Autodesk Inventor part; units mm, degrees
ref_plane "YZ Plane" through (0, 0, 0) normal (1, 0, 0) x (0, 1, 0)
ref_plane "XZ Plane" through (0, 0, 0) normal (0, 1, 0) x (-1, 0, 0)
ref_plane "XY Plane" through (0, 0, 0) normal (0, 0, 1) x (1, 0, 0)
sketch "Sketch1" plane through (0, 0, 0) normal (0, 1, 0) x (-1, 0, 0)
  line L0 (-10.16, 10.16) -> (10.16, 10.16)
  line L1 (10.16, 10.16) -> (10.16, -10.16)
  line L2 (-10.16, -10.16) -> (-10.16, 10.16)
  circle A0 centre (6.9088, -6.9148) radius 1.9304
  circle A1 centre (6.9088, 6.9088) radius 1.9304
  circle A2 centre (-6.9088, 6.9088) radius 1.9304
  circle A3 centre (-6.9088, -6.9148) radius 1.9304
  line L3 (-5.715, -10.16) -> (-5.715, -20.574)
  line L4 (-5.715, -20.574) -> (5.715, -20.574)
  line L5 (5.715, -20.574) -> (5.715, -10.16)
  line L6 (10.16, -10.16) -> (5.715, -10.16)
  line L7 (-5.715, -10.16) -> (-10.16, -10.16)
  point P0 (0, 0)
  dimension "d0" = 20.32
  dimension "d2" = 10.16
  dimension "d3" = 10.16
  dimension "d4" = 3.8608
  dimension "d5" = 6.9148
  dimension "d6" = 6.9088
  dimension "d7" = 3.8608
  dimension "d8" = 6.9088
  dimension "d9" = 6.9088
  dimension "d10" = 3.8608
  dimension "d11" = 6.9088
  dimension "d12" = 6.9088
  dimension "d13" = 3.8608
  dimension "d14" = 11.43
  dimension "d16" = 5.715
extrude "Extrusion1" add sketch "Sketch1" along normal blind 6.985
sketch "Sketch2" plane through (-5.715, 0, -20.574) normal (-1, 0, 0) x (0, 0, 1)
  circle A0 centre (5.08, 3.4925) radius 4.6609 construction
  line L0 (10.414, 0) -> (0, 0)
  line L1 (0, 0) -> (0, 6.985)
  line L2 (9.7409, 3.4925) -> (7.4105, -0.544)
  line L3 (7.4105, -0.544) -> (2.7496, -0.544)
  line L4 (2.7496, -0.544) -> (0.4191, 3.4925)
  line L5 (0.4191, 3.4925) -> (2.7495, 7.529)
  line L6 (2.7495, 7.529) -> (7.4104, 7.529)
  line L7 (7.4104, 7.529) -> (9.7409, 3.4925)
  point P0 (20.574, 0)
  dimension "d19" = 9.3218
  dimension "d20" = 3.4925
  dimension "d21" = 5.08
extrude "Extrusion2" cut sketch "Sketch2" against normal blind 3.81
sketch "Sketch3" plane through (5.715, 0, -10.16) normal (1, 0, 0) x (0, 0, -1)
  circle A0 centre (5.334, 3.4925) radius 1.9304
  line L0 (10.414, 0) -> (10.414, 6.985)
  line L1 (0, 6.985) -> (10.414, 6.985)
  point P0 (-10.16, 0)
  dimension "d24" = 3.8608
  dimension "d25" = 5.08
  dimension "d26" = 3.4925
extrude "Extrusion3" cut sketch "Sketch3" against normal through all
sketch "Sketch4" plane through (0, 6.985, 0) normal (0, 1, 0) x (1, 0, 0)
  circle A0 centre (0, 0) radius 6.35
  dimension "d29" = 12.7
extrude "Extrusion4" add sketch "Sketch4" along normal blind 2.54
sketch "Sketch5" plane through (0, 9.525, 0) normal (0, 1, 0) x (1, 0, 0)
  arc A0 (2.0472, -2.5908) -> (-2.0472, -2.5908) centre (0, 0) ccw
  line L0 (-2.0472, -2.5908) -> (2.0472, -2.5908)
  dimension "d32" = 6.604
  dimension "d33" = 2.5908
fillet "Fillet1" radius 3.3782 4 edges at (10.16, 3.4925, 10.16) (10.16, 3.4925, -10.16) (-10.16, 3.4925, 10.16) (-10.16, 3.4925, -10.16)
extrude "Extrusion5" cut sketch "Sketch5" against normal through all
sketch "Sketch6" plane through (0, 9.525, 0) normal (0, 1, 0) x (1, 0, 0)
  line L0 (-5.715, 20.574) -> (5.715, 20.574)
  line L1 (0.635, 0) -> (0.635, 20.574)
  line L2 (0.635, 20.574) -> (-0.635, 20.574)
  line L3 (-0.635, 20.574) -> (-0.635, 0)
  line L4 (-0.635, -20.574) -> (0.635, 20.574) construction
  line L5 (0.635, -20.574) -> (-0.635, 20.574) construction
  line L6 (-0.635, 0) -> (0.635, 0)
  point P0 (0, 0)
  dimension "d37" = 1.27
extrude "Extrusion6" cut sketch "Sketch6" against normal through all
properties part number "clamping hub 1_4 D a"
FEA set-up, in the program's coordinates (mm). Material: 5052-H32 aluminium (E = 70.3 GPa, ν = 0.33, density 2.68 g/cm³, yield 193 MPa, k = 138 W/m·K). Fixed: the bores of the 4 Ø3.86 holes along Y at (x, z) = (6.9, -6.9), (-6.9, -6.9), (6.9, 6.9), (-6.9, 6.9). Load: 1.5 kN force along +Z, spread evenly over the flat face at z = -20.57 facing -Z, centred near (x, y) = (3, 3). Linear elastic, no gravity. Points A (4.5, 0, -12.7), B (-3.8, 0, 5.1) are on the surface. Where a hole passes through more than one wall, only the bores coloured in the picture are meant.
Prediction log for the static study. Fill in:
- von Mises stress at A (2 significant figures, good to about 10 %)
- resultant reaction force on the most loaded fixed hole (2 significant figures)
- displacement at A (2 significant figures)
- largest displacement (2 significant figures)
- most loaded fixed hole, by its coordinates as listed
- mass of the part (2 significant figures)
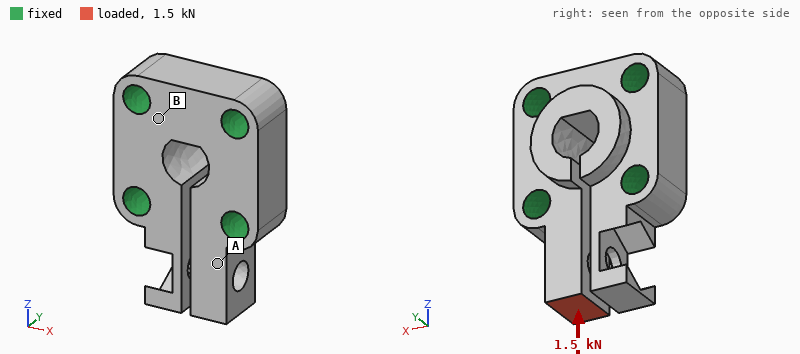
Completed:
81 MPa
1.3 kN
7.2 µm
23 µm
(6.9, -6.9)
7.8 g
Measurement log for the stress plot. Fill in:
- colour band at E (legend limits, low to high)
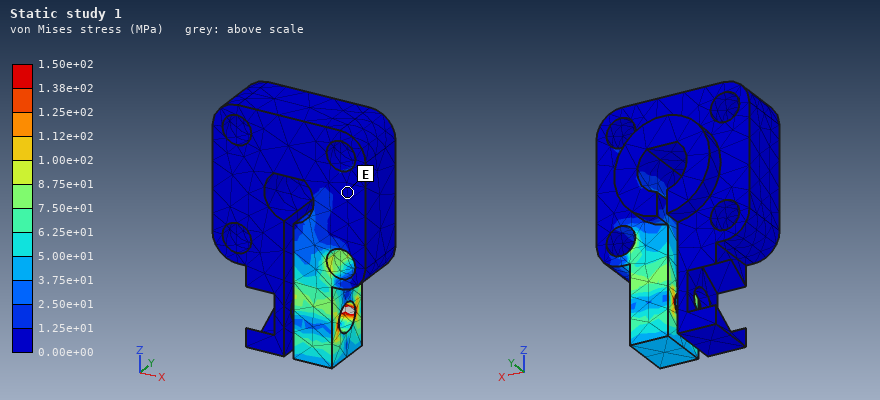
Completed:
0.00e+00 to 1.25e+01 MPa
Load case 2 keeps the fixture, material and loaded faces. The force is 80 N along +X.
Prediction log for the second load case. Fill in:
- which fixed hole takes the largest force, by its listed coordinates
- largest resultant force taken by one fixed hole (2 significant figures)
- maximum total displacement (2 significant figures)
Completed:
(6.9, -6.9)
130 N
16 µm
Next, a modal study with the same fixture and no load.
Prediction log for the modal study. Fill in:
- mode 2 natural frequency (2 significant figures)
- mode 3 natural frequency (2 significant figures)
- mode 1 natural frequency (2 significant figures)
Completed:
14 kHz
22 kHz
6300 Hz
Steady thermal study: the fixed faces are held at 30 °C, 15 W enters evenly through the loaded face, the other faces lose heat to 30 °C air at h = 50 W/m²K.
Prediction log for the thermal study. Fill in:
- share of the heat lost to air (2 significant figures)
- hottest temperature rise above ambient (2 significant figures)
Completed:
3.2 %
53 K
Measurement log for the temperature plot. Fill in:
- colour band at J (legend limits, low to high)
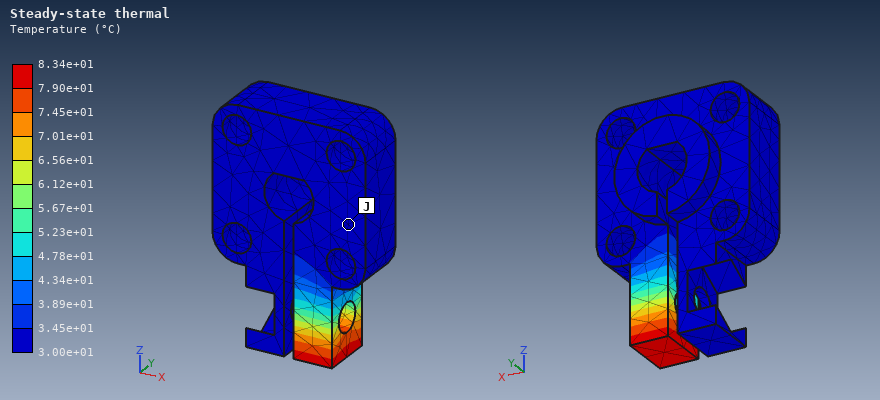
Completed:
3.00e+01 to 3.45e+01 °C
